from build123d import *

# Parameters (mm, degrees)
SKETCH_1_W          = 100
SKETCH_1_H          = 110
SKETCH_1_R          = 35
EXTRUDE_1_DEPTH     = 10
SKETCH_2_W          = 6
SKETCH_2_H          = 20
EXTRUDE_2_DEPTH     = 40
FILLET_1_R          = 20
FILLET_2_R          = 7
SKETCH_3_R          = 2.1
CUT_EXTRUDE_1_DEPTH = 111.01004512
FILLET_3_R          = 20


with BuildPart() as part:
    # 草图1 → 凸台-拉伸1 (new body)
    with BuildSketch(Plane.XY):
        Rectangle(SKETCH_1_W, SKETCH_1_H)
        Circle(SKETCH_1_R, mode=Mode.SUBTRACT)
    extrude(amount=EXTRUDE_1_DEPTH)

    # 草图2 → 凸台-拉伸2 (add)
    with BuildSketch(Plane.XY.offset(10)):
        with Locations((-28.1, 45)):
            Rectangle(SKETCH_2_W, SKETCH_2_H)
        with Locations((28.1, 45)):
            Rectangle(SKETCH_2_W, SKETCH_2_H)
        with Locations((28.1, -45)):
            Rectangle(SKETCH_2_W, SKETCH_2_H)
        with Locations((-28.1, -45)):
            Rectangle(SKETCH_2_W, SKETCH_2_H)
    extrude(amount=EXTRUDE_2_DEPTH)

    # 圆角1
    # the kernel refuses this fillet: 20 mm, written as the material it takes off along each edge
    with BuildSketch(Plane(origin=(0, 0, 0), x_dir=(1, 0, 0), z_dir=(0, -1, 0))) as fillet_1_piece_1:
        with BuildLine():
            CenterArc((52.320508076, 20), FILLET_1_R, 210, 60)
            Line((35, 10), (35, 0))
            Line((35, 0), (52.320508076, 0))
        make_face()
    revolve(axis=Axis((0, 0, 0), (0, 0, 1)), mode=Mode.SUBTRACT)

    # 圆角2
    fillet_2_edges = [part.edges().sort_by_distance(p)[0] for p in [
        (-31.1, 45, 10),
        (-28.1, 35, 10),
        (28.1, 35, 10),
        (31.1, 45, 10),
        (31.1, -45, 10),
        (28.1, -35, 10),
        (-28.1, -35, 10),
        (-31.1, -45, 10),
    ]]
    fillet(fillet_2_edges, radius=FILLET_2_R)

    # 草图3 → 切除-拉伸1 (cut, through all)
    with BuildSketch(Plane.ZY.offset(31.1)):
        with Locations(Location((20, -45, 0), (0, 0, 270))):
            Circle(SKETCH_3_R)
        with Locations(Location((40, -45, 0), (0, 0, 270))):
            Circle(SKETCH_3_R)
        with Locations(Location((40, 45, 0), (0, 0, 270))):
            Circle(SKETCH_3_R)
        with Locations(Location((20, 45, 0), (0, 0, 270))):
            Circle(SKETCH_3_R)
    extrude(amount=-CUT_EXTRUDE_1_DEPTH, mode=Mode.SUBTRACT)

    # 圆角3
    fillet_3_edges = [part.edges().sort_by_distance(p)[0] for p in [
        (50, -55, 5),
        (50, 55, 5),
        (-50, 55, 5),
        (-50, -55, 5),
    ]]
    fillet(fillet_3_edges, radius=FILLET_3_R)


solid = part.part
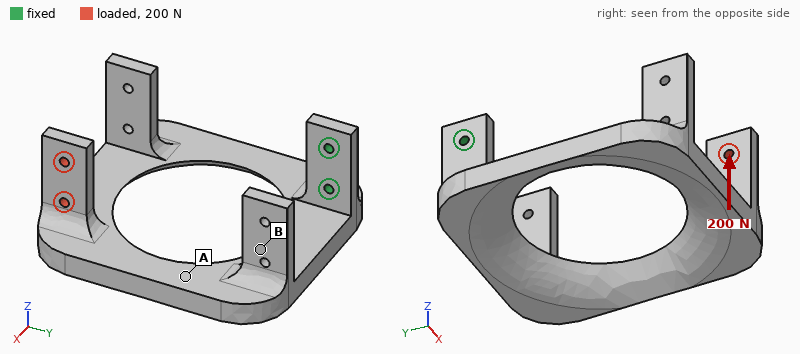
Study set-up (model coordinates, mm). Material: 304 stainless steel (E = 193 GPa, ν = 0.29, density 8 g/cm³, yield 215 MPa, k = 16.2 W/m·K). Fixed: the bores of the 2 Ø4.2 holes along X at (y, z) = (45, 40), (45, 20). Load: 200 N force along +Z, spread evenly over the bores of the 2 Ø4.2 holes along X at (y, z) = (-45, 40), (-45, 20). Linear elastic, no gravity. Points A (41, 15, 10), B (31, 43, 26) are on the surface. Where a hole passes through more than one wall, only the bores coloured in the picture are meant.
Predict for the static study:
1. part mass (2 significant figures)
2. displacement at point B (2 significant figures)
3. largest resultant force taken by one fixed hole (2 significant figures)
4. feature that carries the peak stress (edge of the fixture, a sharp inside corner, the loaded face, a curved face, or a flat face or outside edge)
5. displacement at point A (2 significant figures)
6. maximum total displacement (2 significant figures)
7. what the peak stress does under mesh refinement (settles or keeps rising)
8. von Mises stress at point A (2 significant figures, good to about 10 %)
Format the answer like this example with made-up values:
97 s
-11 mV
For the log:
600 g
0.15 mm
660 N
edge of the fixture
0.23 mm
0.47 mm
keeps rising
22 MPa
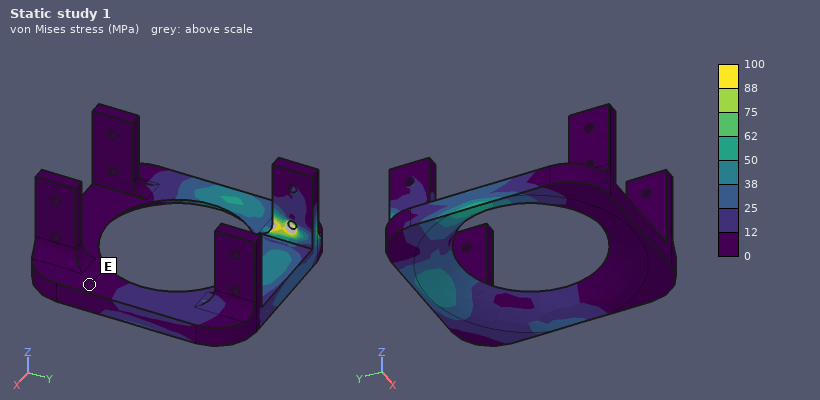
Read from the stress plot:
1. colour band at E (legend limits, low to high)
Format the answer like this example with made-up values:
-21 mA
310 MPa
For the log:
0 to 12 MPa
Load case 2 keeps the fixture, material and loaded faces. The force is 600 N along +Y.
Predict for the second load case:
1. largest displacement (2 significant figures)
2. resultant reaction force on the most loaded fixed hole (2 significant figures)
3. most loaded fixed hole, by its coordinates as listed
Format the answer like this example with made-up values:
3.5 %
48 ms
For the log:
0.51 mm
380 N
(45, 20)
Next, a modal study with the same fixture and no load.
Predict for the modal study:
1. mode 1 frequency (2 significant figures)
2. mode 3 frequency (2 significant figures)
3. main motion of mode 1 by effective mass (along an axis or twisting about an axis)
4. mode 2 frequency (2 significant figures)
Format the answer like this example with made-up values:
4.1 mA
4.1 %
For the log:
250 Hz
450 Hz
along Z
290 Hz
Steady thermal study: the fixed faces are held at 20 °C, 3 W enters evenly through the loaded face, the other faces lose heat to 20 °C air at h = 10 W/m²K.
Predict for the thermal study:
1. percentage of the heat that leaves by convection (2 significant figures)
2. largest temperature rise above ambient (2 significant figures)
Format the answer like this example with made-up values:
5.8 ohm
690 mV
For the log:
92 %
49 K
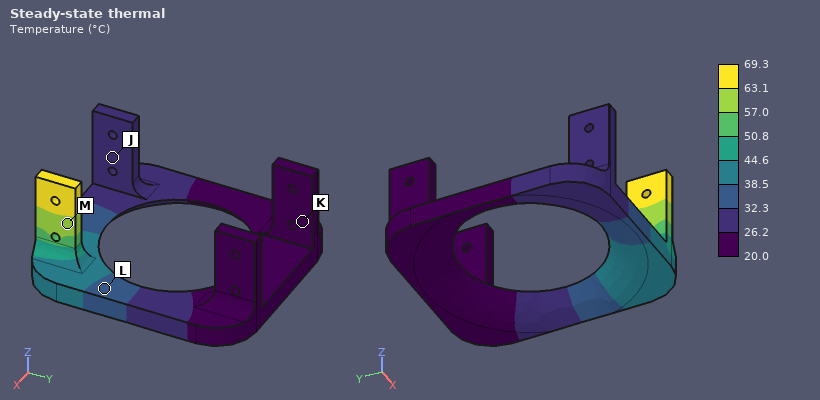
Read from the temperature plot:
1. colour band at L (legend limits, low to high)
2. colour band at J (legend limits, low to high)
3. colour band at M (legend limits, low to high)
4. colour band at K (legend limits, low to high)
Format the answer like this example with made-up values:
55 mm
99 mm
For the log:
32.3 to 38.5 °C
26.2 to 32.3 °C
57.0 to 63.1 °C
20.0 to 26.2 °C
